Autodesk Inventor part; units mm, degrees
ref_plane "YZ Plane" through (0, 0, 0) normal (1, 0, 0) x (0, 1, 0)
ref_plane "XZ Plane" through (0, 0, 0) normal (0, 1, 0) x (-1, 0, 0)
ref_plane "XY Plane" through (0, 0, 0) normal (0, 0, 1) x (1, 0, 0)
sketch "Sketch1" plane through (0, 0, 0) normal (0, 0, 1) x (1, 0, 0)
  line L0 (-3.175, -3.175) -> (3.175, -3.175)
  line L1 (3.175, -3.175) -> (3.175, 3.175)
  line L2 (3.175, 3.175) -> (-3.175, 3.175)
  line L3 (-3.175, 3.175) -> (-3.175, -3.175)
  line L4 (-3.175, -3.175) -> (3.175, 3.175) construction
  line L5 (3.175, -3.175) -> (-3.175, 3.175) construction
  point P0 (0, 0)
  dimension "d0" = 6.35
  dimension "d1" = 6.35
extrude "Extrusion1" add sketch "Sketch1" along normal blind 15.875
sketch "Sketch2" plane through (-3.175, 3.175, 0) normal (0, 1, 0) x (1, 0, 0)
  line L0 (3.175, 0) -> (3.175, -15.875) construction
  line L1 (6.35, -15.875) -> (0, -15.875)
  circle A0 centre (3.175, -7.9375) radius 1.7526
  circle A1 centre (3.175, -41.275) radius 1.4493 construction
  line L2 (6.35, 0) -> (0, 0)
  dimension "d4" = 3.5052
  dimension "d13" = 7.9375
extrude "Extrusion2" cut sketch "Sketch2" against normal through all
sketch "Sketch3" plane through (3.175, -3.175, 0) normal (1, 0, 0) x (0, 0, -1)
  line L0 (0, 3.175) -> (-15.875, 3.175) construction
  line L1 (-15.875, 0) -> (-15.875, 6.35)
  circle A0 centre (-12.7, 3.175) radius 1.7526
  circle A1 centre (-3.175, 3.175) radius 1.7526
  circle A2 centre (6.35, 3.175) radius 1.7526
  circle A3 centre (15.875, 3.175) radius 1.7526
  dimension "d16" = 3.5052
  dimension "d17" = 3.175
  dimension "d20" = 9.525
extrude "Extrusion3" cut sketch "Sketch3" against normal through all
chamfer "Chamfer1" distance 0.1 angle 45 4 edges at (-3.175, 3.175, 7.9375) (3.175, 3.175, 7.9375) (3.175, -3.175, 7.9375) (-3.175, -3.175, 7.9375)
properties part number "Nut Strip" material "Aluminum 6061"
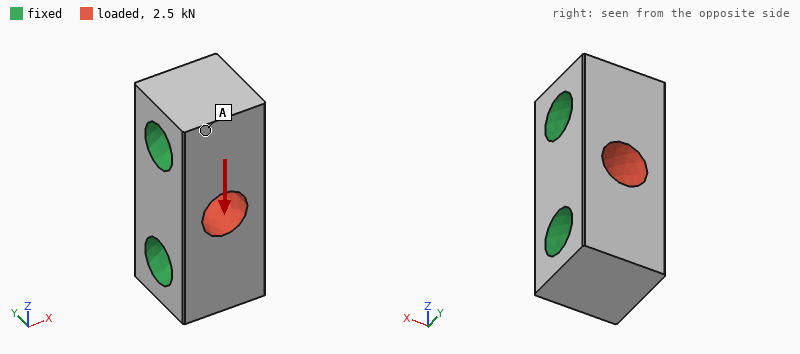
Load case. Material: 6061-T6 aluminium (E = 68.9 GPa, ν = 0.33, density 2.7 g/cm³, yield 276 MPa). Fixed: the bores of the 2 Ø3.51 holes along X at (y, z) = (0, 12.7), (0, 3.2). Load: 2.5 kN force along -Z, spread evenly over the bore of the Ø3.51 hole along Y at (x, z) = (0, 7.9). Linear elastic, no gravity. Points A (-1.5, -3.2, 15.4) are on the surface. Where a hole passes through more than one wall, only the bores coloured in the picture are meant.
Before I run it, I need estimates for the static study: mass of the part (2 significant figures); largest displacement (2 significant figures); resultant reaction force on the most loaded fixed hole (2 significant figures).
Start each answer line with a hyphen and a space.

- 1.2 g
- 1.9 µm
- 1.3 kN
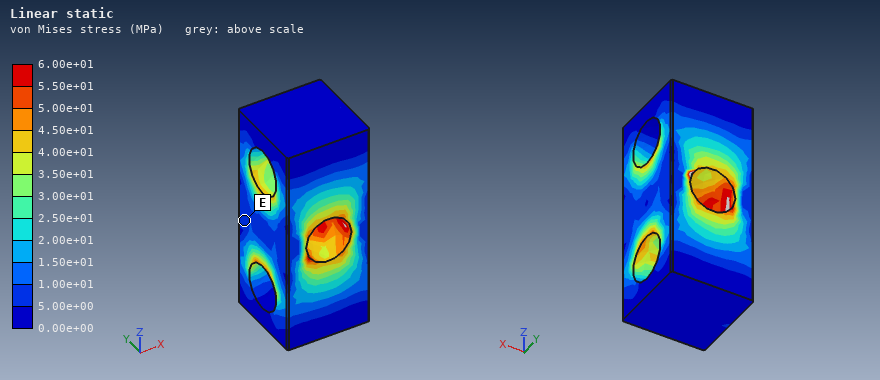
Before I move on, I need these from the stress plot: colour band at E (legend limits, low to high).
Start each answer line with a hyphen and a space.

- 5.00e+00 to 1.00e+01 MPa
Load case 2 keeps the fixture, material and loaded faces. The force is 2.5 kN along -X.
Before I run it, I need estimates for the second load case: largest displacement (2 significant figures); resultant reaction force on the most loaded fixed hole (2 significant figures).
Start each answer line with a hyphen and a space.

- 5.8 µm
- 1.3 kN
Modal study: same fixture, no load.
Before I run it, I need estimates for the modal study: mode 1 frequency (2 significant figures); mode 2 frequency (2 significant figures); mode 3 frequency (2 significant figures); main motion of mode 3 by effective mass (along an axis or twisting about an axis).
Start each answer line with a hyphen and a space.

- 200 kHz
- 210 kHz
- 220 kHz
- along X
